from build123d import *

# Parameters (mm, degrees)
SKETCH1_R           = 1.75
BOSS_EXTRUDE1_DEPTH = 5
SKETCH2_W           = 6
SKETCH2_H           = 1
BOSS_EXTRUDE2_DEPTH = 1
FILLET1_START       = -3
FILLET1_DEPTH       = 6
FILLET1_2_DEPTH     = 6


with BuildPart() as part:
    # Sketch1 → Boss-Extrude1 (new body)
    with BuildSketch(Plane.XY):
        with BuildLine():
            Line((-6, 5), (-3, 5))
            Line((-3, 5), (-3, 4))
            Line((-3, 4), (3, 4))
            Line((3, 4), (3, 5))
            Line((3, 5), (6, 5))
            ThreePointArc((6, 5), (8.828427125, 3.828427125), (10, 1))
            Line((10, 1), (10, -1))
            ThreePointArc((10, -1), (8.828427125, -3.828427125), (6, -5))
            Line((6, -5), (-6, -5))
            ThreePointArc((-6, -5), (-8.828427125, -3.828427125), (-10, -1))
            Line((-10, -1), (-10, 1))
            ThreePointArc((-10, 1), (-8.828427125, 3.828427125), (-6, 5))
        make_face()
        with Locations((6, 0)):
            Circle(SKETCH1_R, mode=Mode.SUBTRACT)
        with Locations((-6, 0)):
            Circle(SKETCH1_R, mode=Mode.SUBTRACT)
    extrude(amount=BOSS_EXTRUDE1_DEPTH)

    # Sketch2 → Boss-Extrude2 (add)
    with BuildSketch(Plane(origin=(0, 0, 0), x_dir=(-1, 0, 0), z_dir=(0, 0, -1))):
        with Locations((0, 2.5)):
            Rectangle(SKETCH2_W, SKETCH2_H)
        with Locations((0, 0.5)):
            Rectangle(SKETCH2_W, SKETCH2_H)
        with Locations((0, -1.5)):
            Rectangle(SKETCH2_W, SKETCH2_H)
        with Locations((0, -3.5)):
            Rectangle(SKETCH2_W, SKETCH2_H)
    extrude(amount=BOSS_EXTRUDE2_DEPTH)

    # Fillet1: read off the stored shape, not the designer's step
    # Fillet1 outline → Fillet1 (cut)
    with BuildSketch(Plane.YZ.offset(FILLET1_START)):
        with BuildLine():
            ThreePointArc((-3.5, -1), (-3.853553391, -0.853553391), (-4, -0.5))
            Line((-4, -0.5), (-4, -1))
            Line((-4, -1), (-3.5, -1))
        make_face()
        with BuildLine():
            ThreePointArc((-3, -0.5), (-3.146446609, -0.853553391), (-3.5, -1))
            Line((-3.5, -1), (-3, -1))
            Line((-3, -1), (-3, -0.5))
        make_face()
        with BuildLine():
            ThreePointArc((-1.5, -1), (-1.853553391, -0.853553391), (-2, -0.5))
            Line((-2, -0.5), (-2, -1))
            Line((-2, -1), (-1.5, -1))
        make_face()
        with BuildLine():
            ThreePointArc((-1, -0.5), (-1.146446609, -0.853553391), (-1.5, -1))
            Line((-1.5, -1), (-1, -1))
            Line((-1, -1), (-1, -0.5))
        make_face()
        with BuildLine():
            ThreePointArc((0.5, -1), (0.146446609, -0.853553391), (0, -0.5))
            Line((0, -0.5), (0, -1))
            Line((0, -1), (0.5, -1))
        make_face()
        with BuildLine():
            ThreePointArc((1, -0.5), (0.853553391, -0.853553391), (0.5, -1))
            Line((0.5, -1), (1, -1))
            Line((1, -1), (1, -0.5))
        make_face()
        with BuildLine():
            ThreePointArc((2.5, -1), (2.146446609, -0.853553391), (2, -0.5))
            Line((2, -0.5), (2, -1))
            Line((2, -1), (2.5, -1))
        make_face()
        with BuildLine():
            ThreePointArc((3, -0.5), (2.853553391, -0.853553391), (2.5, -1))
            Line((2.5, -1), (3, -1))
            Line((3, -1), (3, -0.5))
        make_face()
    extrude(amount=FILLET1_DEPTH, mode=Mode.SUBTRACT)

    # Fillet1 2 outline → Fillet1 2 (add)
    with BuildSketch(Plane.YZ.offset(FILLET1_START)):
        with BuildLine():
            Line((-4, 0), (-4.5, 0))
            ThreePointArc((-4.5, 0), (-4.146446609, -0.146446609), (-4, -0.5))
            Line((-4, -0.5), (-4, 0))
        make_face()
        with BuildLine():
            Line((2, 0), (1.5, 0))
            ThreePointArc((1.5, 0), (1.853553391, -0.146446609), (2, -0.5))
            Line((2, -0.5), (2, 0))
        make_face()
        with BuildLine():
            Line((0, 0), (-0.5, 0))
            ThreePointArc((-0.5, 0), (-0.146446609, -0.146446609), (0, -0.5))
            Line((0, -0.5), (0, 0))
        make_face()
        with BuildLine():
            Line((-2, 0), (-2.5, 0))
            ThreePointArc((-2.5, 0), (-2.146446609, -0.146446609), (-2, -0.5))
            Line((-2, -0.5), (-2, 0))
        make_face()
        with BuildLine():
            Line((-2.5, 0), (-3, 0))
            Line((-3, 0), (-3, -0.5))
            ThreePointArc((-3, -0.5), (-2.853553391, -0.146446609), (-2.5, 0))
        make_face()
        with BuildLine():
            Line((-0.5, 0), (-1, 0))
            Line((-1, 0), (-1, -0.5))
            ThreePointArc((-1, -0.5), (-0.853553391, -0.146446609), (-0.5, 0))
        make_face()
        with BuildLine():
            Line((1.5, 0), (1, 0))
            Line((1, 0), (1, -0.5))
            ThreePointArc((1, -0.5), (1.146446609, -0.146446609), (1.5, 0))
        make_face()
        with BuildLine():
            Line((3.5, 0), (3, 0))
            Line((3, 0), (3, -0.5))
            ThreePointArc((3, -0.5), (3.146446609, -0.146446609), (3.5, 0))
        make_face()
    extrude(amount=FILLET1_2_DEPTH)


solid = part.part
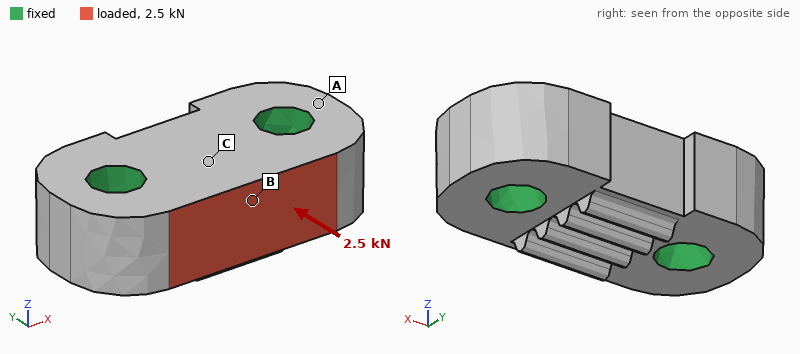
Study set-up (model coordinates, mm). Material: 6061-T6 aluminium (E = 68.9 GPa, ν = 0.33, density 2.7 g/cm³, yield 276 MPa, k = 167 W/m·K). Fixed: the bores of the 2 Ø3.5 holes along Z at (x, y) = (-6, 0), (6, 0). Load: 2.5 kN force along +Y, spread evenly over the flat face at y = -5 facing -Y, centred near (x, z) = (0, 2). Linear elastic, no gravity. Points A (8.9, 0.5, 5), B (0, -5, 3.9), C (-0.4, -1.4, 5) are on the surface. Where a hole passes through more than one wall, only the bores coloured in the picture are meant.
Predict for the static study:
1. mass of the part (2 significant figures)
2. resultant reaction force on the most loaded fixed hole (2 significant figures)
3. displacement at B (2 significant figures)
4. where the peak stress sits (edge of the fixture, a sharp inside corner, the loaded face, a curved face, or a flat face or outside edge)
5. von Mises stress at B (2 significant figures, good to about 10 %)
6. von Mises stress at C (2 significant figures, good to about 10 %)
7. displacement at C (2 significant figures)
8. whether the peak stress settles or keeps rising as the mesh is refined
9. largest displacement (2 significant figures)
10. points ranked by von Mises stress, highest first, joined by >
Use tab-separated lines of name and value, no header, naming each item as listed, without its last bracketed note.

mass of the part	2.2 g
resultant reaction force on the most loaded fixed hole	1.3 kN
displacement at B	4.8 µm
where the peak stress sits	edge of the fixture
von Mises stress at B	43 MPa
von Mises stress at C	23 MPa
displacement at C	3.4 µm
whether the peak stress settles or keeps rising as the mesh is refined	keeps rising
largest displacement	5.0 µm
points ranked by von Mises stress, highest first, joined by >	B > C > A
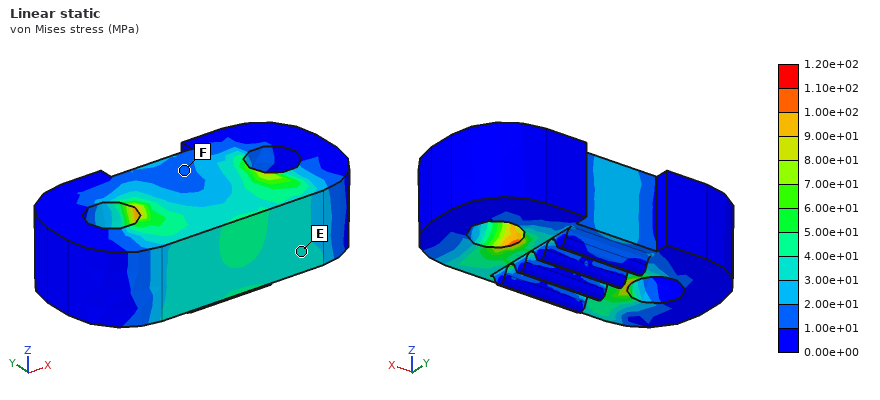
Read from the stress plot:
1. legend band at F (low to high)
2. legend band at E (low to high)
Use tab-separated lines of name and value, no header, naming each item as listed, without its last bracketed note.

legend band at F	1.00e+01 to 2.00e+01 MPa
legend band at E	3.00e+01 to 4.00e+01 MPa
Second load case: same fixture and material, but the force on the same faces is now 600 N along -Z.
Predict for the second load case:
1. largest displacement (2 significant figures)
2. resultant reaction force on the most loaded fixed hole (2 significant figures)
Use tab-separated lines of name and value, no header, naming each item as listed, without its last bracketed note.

largest displacement	5.6 µm
resultant reaction force on the most loaded fixed hole	300 N
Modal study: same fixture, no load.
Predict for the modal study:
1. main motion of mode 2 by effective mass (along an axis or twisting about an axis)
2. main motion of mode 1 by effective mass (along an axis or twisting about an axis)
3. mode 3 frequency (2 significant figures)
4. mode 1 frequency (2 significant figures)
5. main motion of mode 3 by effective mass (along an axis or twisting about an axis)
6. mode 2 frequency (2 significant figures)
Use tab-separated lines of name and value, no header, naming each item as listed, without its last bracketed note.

main motion of mode 2 by effective mass	along Z
main motion of mode 1 by effective mass	along Z
mode 3 frequency	120 kHz
mode 1 frequency	100 kHz
main motion of mode 3 by effective mass	along Y
mode 2 frequency	120 kHz
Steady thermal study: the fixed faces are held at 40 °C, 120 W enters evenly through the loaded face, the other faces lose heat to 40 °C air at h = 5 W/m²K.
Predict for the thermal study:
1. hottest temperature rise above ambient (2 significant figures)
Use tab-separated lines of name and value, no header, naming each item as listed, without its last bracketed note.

hottest temperature rise above ambient	56 K
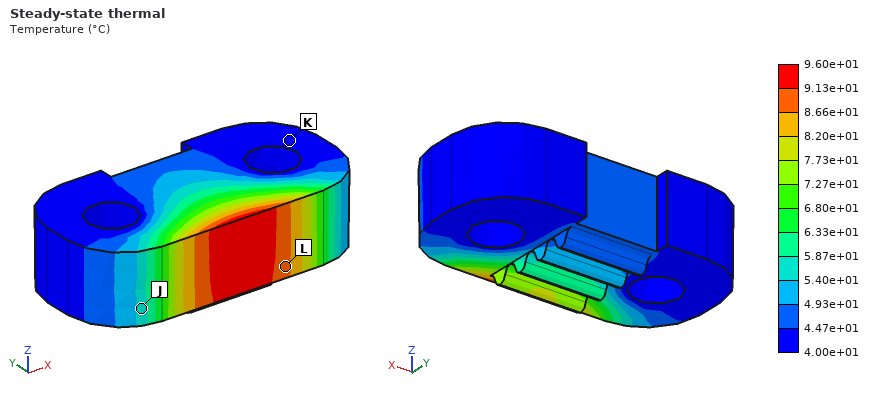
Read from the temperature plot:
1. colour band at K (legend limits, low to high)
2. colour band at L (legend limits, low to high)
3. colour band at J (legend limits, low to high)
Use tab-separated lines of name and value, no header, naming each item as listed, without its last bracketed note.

colour band at K	4.00e+01 to 4.47e+01 °C
colour band at L	8.66e+01 to 9.13e+01 °C
colour band at J	5.40e+01 to 5.87e+01 °C
